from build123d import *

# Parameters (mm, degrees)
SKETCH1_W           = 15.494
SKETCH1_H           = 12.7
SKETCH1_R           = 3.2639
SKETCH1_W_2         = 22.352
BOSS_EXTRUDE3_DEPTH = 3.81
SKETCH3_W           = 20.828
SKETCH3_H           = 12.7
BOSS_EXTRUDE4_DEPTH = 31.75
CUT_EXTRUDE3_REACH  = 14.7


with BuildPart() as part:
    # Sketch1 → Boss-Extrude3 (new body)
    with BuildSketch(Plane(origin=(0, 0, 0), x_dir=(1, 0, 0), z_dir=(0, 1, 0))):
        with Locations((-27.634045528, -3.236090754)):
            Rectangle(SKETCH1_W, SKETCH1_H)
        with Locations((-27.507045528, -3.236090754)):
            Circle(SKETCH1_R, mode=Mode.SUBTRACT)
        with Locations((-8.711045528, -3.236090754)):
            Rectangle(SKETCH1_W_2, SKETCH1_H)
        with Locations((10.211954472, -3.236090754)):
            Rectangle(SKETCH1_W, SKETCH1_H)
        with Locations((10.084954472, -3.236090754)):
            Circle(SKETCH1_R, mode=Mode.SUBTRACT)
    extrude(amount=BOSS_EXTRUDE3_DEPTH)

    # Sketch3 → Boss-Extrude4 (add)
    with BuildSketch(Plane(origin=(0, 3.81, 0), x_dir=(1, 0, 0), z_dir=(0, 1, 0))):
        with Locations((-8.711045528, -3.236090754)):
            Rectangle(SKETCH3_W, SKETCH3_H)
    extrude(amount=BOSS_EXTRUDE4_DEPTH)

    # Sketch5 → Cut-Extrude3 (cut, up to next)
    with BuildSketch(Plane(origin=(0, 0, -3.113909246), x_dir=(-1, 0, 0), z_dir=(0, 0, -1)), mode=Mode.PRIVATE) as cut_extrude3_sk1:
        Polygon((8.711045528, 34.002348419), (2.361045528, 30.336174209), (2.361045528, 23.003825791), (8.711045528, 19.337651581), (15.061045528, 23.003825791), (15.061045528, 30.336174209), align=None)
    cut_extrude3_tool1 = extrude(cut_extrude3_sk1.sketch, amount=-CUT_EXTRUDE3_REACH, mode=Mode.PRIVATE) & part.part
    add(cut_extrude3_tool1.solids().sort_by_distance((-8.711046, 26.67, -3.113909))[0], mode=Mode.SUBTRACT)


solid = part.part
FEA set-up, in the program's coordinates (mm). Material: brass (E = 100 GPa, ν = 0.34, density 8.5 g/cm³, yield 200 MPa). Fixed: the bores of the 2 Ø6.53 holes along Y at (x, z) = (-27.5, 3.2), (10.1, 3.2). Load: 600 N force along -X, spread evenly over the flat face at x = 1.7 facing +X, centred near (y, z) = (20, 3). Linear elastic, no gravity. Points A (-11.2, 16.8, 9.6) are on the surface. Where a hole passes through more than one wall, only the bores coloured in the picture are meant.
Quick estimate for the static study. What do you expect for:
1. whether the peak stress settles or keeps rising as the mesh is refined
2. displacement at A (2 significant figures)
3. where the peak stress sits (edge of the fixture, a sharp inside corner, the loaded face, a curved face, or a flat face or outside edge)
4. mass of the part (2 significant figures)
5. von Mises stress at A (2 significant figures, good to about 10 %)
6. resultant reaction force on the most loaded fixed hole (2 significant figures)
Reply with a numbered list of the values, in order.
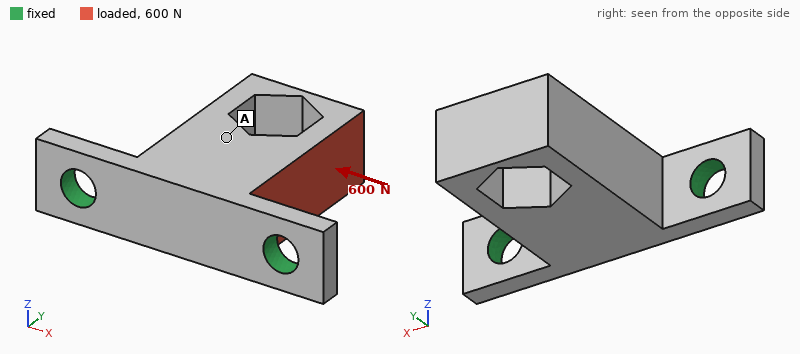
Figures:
1. keeps rising
2. 6.8 µm
3. edge of the fixture
4. 76 g
5. 6.4 MPa
6. 500 N
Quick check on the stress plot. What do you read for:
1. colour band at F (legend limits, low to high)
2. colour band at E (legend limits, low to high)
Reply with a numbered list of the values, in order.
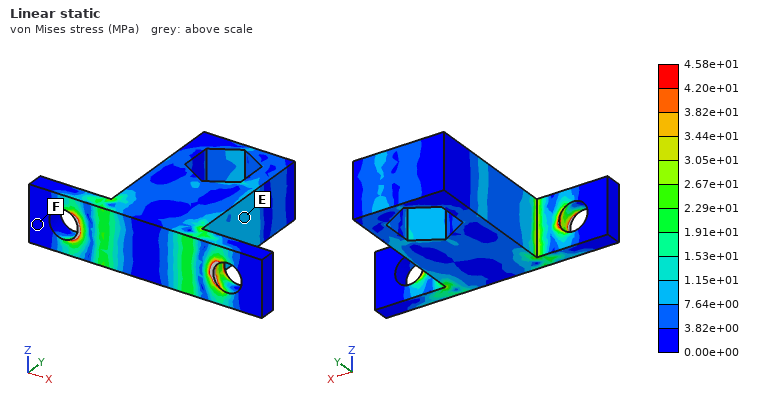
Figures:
1. 0.00e+00 to 3.82e+00 MPa
2. 7.64e+00 to 1.15e+01 MPa
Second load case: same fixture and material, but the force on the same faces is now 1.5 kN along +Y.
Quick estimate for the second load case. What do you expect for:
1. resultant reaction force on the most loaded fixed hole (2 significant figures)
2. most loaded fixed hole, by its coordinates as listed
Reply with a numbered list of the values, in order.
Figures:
1. 1.4 kN
2. (10.1, 3.2)
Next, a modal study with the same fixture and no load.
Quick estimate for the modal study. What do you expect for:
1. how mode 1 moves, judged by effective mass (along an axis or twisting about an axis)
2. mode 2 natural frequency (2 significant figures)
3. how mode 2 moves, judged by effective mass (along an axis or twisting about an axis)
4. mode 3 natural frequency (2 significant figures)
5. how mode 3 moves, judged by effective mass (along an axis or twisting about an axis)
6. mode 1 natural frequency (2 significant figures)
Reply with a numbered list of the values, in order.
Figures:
1. along Z
2. 4900 Hz
3. along X
4. 7600 Hz
5. along Y
6. 1800 Hz
